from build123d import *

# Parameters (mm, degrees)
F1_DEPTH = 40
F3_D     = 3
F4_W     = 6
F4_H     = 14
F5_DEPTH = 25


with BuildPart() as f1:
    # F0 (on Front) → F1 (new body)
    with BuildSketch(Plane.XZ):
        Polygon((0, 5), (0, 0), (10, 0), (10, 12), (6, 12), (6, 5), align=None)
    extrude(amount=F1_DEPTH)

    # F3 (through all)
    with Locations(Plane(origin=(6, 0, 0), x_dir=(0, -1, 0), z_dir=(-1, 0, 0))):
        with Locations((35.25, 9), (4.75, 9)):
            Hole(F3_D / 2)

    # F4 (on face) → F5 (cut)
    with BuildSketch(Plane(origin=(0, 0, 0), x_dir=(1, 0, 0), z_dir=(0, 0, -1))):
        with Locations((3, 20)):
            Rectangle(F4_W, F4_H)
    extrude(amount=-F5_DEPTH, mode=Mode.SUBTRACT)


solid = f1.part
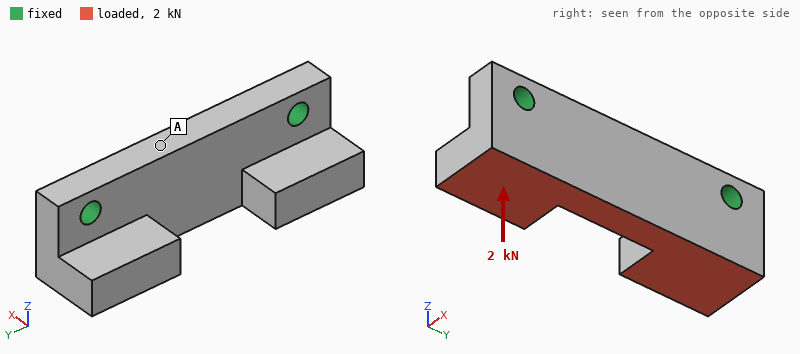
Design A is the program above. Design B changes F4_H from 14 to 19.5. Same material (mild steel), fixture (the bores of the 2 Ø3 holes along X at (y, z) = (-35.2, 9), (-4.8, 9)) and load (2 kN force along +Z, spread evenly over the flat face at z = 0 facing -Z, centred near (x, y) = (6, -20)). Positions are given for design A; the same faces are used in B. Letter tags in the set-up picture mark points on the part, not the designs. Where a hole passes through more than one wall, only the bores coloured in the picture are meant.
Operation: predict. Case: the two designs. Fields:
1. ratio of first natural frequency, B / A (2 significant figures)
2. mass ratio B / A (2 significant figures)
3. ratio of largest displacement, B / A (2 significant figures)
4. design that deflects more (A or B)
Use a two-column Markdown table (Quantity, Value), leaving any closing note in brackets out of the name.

| Quantity | Value |
|---|---|
| ratio of first natural frequency, B / A | 1.1 |
| mass ratio B / A | 0.94 |
| ratio of largest displacement, B / A | 0.88 |
| design that deflects more | A |
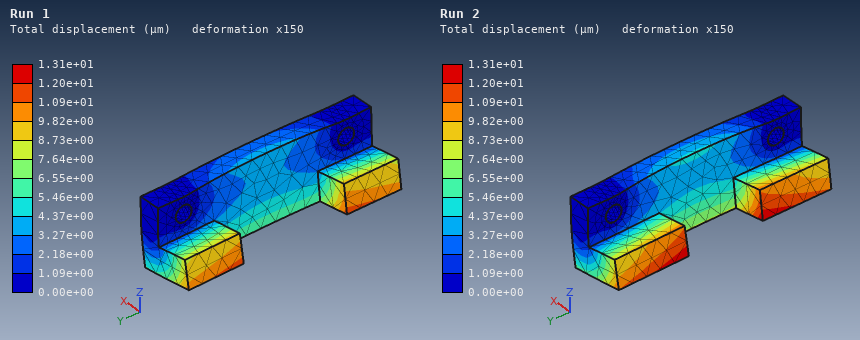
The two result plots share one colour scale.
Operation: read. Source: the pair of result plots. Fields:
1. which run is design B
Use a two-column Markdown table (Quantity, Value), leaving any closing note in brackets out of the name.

| Quantity | Value |
|---|---|
| which run is design B | Run 1 |
